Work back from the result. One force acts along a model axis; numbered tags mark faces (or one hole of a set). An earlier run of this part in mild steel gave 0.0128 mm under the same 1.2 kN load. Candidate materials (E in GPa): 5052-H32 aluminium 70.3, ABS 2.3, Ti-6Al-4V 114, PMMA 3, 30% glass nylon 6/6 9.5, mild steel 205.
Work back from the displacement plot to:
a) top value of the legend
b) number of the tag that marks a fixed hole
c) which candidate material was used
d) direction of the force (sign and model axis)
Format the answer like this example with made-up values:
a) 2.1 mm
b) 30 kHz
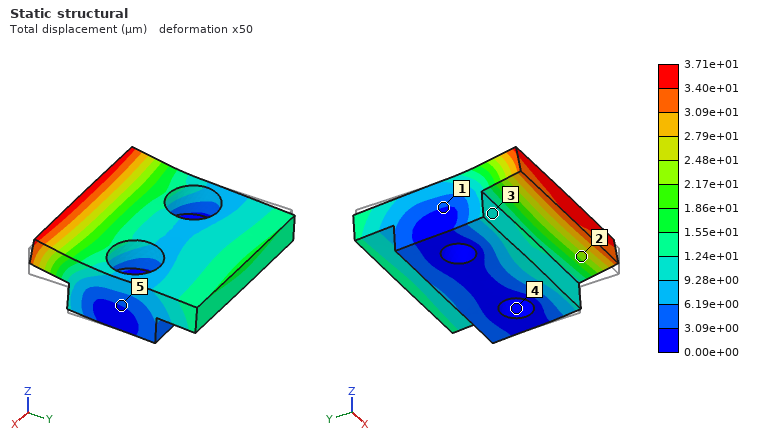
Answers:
a) 3.71e+01 µm
b) 4
c) 5052-H32 aluminium
d) +Z
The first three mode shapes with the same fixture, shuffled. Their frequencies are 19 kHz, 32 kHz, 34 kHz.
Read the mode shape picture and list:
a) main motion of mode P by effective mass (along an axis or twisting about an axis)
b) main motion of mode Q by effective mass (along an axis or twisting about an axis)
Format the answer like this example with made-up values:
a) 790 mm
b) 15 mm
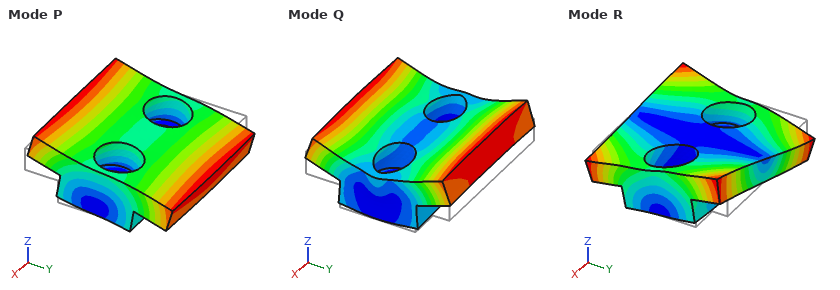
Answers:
a) along Y
b) along Z
